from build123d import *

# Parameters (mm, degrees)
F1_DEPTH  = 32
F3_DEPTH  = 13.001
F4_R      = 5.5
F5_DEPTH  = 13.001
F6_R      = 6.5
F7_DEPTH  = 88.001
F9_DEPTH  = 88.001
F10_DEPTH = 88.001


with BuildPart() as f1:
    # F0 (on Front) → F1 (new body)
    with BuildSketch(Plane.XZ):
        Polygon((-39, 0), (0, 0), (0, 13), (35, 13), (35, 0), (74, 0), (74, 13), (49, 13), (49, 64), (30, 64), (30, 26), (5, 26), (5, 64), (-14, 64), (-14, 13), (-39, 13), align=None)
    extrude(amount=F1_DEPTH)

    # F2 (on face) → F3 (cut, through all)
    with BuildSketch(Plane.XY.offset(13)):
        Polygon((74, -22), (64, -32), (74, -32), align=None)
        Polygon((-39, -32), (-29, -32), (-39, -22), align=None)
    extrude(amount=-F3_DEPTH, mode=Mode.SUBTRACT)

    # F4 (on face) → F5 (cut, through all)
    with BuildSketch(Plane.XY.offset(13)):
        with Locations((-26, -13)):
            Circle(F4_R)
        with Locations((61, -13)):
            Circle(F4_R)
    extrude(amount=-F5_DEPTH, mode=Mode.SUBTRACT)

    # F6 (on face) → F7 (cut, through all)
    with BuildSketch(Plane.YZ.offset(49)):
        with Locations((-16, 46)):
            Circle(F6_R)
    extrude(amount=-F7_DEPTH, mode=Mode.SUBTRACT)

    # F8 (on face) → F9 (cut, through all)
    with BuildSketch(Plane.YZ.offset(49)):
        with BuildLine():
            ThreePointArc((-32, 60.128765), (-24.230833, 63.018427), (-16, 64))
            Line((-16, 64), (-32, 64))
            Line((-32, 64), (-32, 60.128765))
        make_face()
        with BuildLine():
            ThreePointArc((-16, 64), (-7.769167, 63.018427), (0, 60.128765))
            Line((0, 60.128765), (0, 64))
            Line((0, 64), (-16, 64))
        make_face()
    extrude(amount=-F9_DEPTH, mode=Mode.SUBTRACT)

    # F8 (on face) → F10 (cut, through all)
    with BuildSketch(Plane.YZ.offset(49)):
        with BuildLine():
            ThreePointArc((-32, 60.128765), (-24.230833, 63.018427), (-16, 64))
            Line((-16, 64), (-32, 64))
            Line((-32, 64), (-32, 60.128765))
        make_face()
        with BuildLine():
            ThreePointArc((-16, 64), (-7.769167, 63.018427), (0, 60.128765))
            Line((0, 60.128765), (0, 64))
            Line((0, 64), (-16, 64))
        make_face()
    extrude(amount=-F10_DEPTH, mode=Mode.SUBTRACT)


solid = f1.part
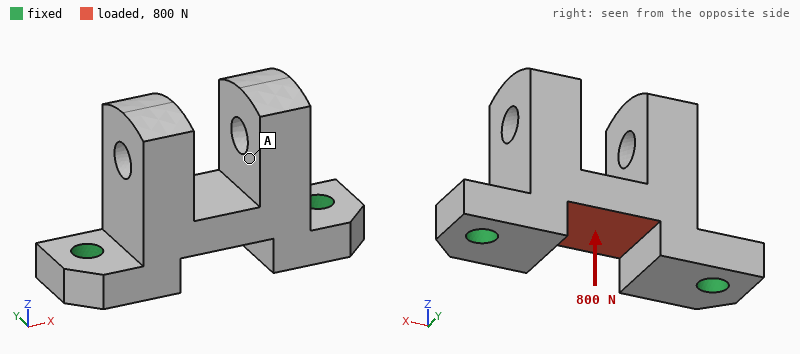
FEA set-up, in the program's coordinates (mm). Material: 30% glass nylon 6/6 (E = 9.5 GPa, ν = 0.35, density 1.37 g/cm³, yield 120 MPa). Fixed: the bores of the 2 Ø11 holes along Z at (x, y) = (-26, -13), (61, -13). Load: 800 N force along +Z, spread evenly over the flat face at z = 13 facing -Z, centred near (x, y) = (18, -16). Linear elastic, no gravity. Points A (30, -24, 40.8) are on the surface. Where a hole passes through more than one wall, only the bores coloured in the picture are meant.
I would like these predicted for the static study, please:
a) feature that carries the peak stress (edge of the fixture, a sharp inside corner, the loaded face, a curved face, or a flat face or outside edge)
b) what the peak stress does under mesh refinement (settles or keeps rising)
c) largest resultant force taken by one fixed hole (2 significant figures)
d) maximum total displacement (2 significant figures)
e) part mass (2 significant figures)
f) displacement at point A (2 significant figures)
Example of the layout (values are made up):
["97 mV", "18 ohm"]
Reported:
["edge of the fixture", "keeps rising", "620 N", "34 µm", "130 g", "24 µm"]
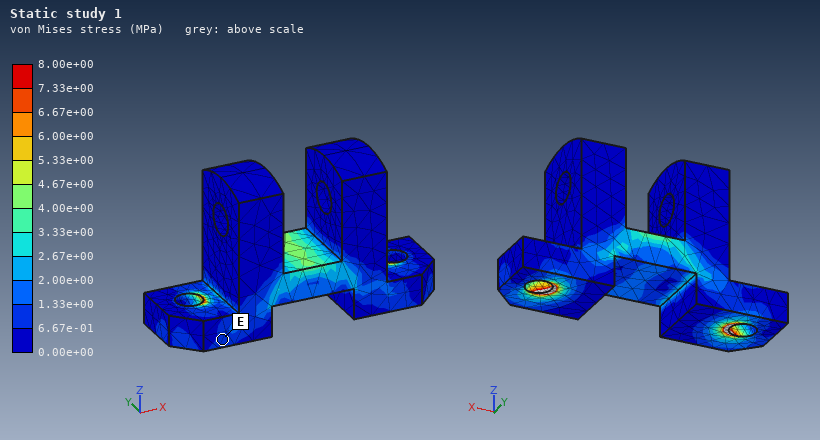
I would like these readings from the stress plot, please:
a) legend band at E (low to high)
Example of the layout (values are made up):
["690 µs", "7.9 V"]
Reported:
["6.67e-01 to 1.33e+00 MPa"]
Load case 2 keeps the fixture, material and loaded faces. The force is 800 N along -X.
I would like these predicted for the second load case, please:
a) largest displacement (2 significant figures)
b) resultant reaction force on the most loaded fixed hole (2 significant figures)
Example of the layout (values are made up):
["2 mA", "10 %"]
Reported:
["13 µm", "400 N"]
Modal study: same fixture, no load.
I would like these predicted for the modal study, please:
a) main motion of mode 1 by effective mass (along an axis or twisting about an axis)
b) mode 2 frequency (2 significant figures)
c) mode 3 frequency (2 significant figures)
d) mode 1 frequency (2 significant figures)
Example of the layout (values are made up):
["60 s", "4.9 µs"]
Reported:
["along Y", "2300 Hz", "2600 Hz", "1500 Hz"]
